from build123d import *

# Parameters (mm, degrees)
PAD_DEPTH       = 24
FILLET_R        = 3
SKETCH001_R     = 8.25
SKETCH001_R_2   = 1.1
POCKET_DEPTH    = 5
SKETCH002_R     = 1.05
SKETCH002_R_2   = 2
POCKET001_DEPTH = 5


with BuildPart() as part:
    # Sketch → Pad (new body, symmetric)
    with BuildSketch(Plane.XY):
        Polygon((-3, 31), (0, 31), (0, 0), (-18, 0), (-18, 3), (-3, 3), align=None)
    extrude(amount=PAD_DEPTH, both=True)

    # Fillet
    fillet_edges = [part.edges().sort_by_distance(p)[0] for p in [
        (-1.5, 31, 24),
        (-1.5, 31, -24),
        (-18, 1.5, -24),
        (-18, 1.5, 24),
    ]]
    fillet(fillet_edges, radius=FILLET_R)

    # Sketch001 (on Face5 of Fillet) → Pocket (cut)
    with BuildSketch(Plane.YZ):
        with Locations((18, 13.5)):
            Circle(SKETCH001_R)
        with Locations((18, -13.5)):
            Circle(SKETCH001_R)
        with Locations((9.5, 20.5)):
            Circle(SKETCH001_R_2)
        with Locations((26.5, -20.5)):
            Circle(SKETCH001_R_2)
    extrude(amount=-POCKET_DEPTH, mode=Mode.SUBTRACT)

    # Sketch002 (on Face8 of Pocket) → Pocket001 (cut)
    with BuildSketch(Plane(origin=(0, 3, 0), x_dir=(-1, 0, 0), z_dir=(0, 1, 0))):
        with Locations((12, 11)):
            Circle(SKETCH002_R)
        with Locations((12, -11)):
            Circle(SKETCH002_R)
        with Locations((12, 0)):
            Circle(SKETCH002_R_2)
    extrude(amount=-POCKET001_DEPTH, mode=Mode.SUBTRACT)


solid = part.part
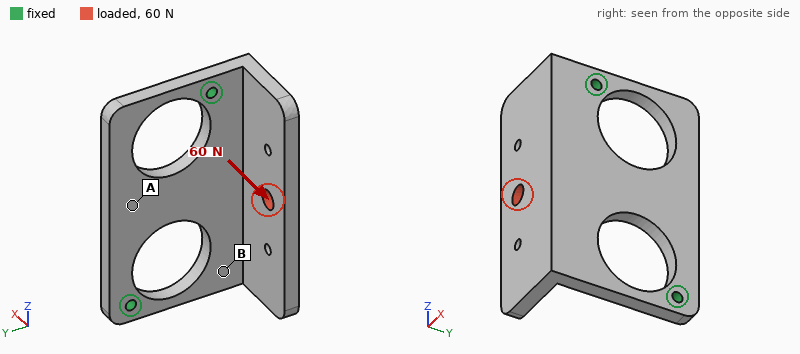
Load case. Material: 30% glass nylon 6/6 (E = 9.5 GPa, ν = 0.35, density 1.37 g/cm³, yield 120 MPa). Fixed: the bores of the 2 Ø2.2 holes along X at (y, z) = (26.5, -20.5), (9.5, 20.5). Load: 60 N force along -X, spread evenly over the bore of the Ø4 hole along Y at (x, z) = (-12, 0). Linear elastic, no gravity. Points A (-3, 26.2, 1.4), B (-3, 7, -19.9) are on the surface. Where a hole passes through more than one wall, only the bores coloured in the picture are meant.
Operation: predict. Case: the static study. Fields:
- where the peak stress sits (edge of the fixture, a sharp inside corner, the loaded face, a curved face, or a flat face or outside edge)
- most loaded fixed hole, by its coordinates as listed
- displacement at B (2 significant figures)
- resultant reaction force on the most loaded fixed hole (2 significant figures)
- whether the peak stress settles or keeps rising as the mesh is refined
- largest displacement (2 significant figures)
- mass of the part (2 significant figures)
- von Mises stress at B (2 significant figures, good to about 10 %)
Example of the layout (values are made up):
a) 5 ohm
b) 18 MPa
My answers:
a) edge of the fixture
b) (9.5, 20.5)
c) 0.33 mm
d) 42 N
e) keeps rising
f) 0.61 mm
g) 7.2 g
h) 10 MPa
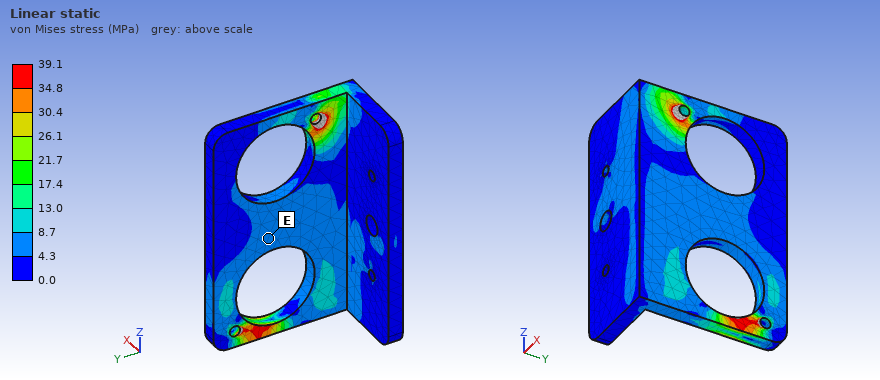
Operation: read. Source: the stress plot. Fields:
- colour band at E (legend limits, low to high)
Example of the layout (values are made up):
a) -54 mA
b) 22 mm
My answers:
a) 4.3 to 8.7 MPa
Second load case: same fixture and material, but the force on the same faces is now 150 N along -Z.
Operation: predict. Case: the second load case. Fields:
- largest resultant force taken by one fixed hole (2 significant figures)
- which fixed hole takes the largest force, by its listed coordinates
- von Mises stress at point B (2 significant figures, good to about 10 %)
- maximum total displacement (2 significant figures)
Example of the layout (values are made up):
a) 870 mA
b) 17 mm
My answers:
a) 140 N
b) (9.5, 20.5)
c) 16 MPa
d) 0.67 mm
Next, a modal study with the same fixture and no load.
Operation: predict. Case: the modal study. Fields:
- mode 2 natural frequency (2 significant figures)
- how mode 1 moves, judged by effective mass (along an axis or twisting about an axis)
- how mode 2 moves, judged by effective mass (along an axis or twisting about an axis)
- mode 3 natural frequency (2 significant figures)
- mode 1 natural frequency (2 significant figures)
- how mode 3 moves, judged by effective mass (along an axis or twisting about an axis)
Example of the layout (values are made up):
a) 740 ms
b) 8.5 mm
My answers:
a) 2000 Hz
b) along X
c) along X
d) 2600 Hz
e) 910 Hz
f) along Y
